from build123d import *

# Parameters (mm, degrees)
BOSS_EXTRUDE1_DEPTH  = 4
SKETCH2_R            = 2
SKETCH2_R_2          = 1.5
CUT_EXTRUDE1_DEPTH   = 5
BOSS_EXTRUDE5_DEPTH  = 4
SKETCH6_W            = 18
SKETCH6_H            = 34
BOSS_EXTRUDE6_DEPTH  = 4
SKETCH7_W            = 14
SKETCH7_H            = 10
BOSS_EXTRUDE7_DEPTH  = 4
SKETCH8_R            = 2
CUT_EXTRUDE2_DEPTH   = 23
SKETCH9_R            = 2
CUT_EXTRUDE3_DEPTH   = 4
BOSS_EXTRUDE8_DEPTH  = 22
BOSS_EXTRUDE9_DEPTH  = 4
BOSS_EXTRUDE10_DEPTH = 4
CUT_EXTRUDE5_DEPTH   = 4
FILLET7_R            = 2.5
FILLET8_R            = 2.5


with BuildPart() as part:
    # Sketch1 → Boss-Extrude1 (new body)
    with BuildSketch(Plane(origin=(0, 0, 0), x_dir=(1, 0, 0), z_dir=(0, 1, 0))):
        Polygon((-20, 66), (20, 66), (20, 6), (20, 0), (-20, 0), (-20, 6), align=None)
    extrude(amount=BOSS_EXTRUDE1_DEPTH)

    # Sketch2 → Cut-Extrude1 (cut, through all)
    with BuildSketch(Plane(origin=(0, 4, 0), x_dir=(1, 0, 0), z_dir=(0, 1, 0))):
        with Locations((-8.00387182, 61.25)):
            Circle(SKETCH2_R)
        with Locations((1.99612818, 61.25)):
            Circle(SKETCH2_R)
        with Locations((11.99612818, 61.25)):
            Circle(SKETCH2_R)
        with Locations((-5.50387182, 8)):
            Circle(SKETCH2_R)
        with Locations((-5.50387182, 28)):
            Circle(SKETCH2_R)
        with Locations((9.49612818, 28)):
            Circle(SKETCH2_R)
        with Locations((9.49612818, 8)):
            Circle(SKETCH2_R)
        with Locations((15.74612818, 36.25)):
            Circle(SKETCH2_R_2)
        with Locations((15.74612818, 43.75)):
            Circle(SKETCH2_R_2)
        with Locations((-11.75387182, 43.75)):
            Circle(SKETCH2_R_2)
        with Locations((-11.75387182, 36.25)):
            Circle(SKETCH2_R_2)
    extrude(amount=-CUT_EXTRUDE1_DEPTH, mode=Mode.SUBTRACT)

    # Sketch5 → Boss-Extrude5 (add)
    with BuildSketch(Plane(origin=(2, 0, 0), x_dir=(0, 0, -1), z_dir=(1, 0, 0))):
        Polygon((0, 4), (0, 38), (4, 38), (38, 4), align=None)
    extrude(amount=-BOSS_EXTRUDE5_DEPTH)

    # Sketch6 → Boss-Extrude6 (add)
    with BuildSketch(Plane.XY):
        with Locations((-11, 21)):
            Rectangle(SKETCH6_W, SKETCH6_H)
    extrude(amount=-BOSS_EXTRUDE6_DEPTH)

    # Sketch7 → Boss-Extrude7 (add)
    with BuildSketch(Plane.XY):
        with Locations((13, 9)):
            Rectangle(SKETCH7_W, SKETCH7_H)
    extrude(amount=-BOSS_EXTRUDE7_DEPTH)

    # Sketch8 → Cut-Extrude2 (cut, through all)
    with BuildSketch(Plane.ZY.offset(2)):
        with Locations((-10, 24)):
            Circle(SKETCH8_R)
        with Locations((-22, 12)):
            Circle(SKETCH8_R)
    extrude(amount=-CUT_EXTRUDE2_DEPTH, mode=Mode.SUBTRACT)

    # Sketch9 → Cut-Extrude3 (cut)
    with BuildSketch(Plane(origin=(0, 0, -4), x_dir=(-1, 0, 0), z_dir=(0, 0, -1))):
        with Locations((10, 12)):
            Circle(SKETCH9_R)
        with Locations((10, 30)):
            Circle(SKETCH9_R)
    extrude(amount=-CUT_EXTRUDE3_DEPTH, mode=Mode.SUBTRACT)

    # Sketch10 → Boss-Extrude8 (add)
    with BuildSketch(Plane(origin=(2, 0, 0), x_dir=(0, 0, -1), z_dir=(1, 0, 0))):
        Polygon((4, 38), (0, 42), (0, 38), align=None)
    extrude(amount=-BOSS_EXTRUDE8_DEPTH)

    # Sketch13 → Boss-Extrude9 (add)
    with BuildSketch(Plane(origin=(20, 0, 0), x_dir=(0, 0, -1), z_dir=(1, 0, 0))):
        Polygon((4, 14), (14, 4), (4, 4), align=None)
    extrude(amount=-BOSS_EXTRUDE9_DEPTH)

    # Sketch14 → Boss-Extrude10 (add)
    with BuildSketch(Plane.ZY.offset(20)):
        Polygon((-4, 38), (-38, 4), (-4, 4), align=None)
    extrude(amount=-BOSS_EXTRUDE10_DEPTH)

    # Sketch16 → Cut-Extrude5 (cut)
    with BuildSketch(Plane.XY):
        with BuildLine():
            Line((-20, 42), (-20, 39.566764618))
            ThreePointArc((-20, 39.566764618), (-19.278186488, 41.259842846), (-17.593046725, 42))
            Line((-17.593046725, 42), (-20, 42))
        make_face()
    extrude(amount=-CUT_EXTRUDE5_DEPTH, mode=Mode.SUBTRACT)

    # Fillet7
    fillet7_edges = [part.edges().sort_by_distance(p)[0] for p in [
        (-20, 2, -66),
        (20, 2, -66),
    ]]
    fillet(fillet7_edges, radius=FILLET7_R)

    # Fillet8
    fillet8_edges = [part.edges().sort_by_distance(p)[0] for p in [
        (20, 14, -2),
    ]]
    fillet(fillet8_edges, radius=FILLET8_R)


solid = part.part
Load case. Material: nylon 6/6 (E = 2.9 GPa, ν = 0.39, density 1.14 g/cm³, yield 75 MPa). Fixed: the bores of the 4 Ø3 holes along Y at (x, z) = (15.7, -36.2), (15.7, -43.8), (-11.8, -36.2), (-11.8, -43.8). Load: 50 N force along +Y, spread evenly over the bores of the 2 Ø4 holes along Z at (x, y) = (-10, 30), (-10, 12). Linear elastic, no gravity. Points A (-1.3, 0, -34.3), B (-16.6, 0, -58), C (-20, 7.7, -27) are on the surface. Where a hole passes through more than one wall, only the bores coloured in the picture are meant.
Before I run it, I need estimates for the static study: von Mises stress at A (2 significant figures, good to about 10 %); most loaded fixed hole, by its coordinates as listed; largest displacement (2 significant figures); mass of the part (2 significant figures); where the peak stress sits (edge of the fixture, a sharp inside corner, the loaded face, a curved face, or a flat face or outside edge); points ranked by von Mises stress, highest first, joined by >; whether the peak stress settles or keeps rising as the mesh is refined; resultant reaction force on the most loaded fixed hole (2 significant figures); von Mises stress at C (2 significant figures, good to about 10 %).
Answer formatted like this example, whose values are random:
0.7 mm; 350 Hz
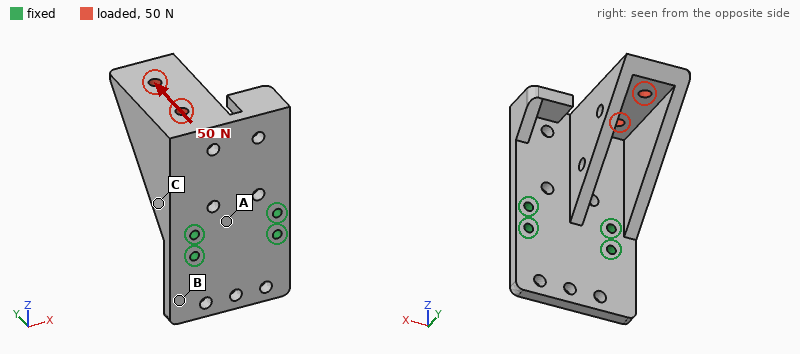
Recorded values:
6.7 MPa; (-11.8, -36.2); 0.92 mm; 21 g; edge of the fixture; A > C > B; keeps rising; 120 N; 2.8 MPa
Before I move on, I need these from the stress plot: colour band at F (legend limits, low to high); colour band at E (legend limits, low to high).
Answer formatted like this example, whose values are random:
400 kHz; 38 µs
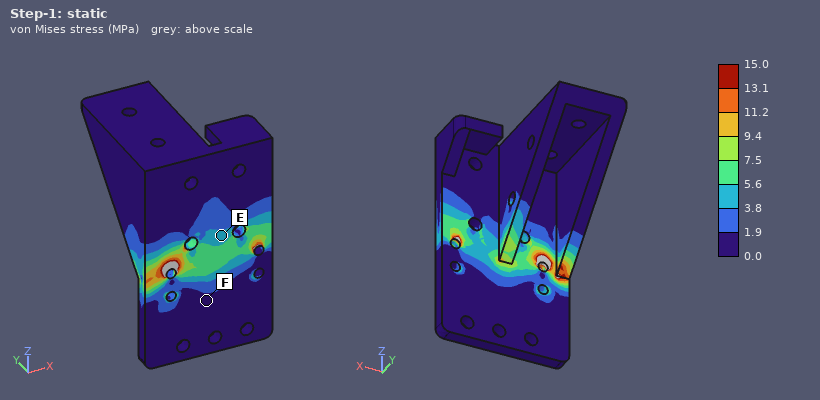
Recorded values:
0.0 to 1.9 MPa; 3.8 to 5.6 MPa
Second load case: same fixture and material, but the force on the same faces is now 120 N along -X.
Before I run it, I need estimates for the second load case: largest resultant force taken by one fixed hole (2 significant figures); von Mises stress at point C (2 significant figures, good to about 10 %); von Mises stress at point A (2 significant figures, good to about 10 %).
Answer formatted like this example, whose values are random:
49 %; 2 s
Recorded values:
140 N; 7.1 MPa; 2.5 MPa
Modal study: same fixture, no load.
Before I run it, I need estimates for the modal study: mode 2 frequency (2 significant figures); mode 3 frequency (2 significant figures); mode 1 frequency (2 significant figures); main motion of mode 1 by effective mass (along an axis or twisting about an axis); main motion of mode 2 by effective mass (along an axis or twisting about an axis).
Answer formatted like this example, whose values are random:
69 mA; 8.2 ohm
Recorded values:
770 Hz; 2000 Hz; 460 Hz; along Y; along X
